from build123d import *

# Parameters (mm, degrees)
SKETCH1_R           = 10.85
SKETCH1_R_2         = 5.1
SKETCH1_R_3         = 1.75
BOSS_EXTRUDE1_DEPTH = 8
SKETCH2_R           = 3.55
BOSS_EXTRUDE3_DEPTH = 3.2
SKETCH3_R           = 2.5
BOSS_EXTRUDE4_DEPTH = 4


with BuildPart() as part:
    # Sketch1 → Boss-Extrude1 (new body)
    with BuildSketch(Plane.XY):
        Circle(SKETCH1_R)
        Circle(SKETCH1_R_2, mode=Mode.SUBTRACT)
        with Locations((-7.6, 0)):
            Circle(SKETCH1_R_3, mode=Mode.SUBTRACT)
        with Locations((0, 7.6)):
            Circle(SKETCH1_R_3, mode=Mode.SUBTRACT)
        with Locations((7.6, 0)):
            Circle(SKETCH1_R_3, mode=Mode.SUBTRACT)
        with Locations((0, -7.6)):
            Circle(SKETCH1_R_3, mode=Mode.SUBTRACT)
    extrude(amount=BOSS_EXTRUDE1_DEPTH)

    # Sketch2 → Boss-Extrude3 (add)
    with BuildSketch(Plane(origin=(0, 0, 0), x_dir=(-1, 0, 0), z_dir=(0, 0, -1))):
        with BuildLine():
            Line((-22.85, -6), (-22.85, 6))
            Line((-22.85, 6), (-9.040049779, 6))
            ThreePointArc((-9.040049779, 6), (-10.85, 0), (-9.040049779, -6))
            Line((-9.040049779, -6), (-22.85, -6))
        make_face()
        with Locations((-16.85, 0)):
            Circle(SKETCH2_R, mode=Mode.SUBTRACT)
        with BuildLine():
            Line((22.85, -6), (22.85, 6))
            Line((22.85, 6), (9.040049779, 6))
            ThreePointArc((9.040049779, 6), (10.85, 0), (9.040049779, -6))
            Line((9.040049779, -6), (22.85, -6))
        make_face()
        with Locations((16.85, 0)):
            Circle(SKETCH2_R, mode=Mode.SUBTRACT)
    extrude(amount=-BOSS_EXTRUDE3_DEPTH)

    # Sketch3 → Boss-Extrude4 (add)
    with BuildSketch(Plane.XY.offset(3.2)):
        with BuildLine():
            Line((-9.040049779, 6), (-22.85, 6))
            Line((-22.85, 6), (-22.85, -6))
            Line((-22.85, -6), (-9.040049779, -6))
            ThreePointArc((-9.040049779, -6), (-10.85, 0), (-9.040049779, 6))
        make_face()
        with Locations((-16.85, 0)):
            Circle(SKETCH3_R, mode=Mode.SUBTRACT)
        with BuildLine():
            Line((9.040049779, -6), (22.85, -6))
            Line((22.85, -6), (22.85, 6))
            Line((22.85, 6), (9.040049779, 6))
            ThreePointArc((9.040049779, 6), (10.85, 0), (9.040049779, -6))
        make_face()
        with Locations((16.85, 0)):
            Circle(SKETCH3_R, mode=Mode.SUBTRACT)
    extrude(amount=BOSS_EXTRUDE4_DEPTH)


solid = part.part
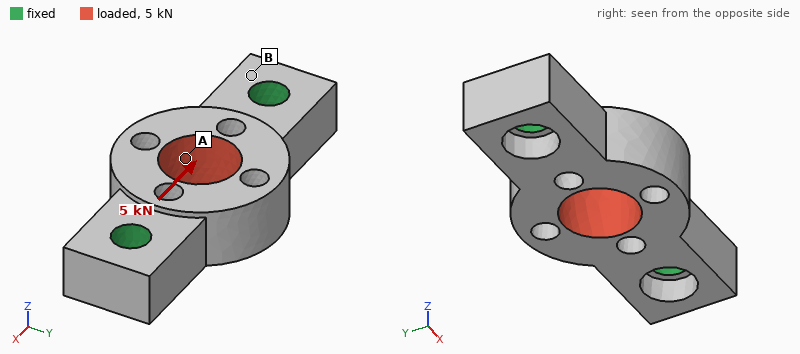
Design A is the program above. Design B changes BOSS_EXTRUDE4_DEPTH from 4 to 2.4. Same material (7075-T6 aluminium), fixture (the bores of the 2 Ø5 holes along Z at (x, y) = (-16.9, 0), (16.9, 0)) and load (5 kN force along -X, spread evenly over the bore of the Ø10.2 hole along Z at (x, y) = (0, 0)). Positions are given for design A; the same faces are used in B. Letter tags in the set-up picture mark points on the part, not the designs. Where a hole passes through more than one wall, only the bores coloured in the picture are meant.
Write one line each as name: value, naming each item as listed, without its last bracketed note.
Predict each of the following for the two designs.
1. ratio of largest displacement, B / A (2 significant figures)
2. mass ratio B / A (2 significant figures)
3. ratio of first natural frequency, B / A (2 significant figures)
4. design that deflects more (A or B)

ratio of largest displacement, B / A: 1.5
mass ratio B / A: 0.89
ratio of first natural frequency, B / A: 0.75
design that deflects more: B
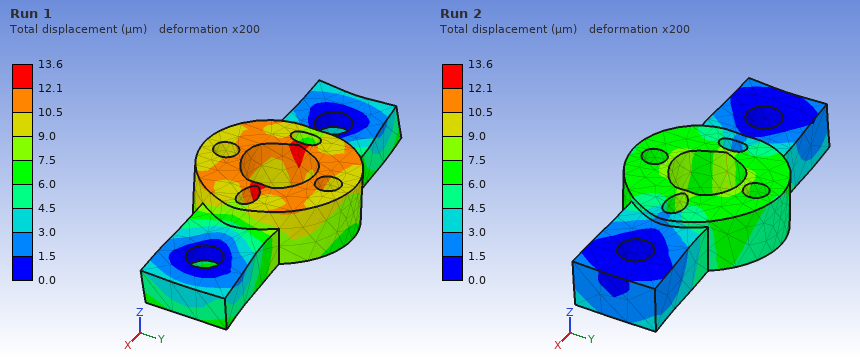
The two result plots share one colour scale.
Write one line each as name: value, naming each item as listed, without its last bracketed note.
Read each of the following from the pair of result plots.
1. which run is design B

which run is design B: Run 1
